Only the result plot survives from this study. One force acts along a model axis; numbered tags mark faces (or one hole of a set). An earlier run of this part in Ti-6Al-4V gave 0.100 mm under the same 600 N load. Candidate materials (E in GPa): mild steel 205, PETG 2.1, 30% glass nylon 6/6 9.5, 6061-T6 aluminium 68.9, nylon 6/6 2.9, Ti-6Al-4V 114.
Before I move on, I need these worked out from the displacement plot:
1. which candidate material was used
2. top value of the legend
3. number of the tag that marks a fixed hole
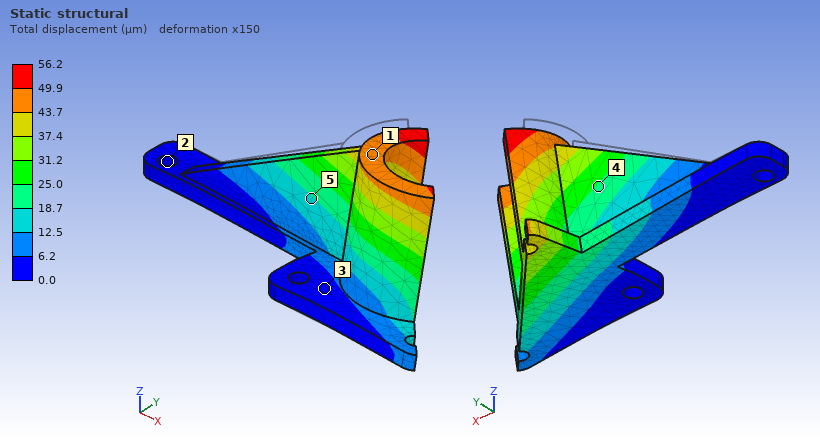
mild steel
56.2 µm
2
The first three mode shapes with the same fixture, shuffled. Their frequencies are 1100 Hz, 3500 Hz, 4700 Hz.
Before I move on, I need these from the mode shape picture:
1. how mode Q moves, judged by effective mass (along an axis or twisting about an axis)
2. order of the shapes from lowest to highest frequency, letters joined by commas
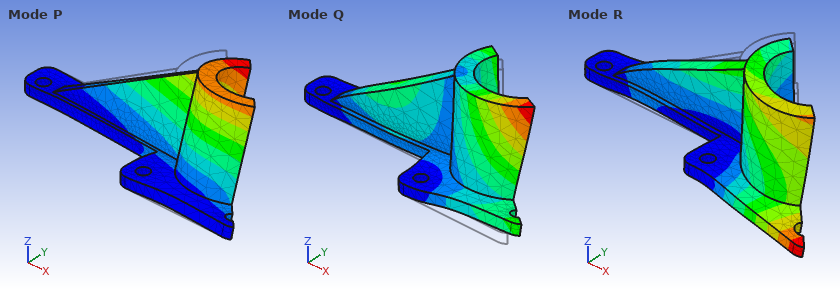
along Z
P, R, Q
